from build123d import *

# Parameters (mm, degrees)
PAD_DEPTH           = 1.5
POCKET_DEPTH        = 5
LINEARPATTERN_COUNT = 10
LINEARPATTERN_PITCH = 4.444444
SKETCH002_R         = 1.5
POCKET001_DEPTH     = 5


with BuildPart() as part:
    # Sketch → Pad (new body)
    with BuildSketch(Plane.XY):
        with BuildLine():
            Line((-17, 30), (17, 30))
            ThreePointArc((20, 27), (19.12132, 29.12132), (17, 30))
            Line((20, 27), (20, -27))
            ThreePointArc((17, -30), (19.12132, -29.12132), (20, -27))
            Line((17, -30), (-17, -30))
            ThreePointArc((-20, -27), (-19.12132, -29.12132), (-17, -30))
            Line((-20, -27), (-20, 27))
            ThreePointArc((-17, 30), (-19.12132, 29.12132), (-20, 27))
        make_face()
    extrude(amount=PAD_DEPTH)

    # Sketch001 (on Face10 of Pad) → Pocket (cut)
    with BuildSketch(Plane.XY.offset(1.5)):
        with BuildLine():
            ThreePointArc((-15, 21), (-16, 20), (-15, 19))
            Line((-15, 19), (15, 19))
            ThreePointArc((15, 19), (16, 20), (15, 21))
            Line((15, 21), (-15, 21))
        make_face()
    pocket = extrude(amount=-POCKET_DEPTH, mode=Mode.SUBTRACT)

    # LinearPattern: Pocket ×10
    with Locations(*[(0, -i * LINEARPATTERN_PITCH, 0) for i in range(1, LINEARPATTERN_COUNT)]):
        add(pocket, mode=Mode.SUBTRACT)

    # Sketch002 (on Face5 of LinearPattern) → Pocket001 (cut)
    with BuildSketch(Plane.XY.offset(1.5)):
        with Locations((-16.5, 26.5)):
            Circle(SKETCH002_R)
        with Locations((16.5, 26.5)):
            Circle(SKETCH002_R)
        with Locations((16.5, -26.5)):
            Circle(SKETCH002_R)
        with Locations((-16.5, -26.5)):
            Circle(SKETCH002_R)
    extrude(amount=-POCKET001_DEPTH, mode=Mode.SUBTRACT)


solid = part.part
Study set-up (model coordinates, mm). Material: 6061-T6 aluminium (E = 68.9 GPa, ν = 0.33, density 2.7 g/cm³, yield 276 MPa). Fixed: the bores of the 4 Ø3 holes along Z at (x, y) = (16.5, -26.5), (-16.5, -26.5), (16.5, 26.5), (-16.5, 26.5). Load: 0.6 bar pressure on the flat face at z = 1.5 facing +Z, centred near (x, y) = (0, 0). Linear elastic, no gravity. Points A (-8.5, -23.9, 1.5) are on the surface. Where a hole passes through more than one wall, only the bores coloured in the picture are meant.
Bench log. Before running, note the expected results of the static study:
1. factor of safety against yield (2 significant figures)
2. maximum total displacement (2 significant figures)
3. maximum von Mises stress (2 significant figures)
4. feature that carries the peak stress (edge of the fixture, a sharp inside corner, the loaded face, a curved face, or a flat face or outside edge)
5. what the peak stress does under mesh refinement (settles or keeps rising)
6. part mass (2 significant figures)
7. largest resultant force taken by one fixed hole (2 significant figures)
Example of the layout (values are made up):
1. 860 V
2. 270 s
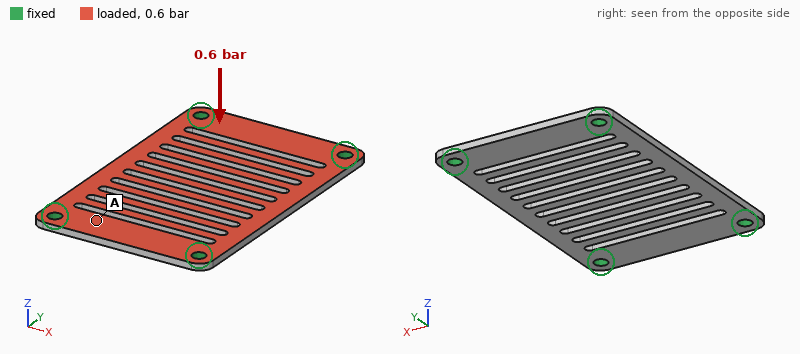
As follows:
1. 2.8
2. 0.18 mm
3. 98 MPa
4. the loaded face
5. settles
6. 7.0 g
7. 26 N
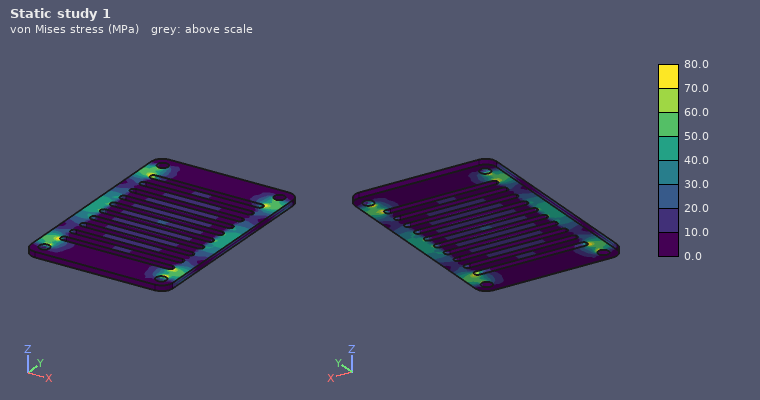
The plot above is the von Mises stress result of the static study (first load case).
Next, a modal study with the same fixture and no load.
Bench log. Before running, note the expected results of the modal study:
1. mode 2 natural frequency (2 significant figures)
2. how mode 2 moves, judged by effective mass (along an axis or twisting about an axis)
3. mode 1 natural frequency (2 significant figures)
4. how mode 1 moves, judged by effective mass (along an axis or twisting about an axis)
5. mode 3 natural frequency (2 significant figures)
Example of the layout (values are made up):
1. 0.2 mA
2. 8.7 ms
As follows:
1. 3200 Hz
2. twisting about Y
3. 1700 Hz
4. along Z
5. 3600 Hz
